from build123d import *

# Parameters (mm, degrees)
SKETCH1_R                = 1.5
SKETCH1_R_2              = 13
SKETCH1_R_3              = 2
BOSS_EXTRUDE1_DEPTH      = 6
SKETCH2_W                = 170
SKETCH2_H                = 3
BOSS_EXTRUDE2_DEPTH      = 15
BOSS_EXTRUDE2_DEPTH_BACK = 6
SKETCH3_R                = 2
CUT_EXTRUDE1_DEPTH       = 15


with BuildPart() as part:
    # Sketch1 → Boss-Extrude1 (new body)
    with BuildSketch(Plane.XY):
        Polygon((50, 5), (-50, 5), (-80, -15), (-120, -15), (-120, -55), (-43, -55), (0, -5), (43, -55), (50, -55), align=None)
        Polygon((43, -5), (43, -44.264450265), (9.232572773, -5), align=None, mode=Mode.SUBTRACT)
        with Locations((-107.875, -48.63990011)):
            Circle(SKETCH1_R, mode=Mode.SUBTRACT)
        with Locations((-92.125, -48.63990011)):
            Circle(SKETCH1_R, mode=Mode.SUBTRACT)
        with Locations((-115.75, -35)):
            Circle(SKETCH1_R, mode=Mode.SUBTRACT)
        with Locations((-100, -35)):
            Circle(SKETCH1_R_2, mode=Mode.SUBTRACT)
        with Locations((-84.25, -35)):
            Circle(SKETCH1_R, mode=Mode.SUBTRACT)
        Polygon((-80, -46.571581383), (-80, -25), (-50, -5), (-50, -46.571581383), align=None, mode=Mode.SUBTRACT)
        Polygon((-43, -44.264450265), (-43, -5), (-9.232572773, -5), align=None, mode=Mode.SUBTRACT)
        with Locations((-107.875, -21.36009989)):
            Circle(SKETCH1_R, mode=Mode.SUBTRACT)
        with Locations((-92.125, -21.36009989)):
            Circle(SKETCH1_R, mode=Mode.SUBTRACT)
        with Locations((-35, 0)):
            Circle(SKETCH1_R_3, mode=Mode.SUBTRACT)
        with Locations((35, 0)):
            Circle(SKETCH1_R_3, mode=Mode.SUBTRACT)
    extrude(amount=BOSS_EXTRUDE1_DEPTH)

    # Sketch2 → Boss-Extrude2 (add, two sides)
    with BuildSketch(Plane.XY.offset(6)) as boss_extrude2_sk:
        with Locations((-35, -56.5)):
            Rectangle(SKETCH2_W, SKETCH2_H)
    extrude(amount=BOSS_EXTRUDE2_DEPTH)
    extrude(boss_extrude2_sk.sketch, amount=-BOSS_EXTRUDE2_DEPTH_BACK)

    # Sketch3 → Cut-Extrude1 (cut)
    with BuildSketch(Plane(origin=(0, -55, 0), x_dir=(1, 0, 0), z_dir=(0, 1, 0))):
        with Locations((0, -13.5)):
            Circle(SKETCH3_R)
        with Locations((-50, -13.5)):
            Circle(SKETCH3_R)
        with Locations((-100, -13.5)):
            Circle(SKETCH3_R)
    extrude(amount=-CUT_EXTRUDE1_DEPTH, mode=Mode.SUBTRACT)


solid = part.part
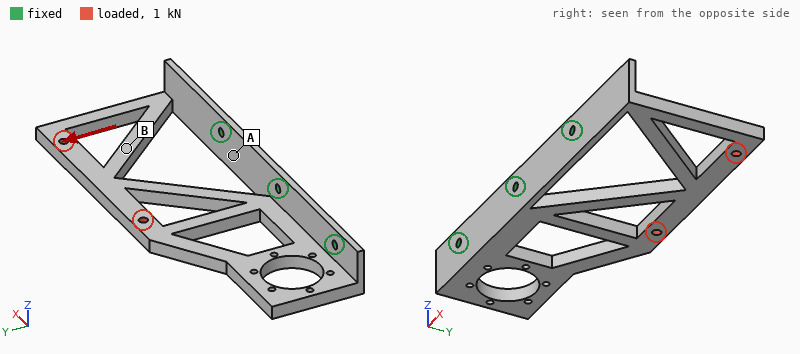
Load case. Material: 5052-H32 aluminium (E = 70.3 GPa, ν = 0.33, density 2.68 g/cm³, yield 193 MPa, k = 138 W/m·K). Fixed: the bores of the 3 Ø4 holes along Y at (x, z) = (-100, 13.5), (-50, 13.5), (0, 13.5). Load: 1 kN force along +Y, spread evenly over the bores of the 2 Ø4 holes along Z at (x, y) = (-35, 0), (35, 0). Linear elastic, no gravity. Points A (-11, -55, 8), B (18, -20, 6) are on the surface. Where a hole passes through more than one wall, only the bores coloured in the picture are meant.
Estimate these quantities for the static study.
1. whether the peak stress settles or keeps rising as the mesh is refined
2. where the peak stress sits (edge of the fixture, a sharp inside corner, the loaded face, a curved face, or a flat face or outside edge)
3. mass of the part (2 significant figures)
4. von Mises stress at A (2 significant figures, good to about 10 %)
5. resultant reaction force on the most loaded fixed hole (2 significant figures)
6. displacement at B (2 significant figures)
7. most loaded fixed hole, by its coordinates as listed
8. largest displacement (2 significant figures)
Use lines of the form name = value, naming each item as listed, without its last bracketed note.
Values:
whether the peak stress settles or keeps rising as the mesh is refined = keeps rising
where the peak stress sits = edge of the fixture
mass of the part = 94 g
von Mises stress at A = 30 MPa
resultant reaction force on the most loaded fixed hole = 1.6 kN
displacement at B = 0.47 mm
most loaded fixed hole, by its coordinates as listed = (-50, 13.5)
largest displacement = 0.76 mm
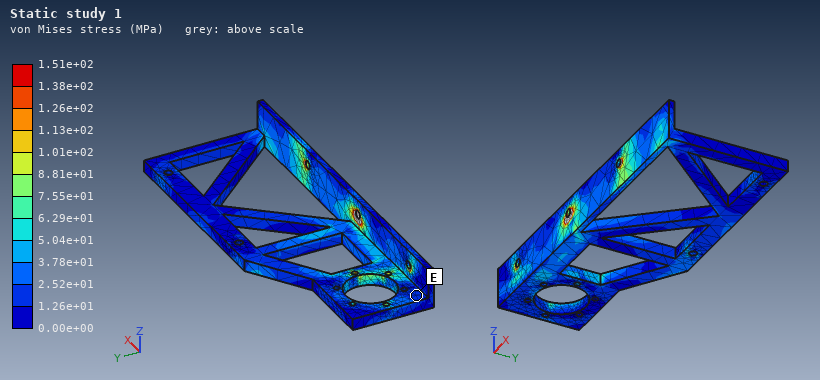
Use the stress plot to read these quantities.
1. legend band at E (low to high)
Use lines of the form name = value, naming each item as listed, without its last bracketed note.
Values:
legend band at E = 1.26e+01 to 2.52e+01 MPa
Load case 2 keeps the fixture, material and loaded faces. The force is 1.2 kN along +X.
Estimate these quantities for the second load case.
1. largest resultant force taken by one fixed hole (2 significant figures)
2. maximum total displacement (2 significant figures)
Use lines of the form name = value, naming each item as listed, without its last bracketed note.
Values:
largest resultant force taken by one fixed hole = 1.3 kN
maximum total displacement = 0.54 mm
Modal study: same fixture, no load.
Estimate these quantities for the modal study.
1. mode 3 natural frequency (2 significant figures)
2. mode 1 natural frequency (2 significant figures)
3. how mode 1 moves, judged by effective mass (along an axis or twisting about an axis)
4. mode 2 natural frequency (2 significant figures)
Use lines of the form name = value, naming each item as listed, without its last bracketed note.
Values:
mode 3 natural frequency = 1100 Hz
mode 1 natural frequency = 400 Hz
how mode 1 moves, judged by effective mass = along Z
mode 2 natural frequency = 1000 Hz
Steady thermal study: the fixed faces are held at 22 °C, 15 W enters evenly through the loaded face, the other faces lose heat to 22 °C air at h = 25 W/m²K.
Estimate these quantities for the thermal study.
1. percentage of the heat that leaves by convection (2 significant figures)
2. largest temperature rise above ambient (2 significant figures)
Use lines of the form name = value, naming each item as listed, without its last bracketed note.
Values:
percentage of the heat that leaves by convection = 46 %
largest temperature rise above ambient = 42 K
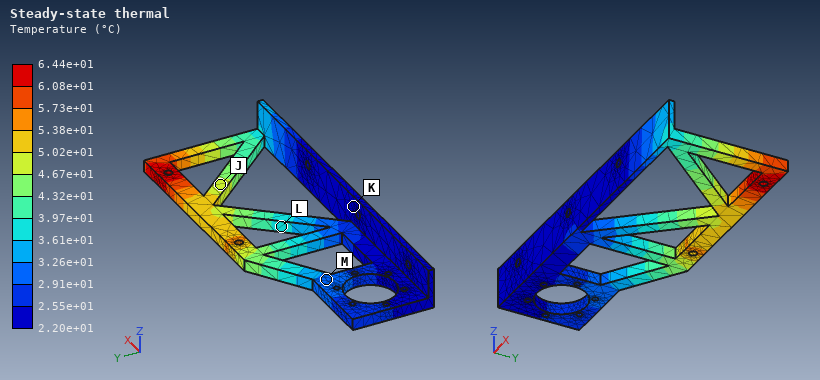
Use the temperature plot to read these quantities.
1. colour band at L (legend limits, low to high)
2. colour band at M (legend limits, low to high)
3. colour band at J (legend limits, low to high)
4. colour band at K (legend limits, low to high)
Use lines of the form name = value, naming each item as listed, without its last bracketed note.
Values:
colour band at L = 3.61e+01 to 3.97e+01 °C
colour band at M = 2.91e+01 to 3.26e+01 °C
colour band at J = 4.67e+01 to 5.02e+01 °C
colour band at K = 2.20e+01 to 2.55e+01 °C
